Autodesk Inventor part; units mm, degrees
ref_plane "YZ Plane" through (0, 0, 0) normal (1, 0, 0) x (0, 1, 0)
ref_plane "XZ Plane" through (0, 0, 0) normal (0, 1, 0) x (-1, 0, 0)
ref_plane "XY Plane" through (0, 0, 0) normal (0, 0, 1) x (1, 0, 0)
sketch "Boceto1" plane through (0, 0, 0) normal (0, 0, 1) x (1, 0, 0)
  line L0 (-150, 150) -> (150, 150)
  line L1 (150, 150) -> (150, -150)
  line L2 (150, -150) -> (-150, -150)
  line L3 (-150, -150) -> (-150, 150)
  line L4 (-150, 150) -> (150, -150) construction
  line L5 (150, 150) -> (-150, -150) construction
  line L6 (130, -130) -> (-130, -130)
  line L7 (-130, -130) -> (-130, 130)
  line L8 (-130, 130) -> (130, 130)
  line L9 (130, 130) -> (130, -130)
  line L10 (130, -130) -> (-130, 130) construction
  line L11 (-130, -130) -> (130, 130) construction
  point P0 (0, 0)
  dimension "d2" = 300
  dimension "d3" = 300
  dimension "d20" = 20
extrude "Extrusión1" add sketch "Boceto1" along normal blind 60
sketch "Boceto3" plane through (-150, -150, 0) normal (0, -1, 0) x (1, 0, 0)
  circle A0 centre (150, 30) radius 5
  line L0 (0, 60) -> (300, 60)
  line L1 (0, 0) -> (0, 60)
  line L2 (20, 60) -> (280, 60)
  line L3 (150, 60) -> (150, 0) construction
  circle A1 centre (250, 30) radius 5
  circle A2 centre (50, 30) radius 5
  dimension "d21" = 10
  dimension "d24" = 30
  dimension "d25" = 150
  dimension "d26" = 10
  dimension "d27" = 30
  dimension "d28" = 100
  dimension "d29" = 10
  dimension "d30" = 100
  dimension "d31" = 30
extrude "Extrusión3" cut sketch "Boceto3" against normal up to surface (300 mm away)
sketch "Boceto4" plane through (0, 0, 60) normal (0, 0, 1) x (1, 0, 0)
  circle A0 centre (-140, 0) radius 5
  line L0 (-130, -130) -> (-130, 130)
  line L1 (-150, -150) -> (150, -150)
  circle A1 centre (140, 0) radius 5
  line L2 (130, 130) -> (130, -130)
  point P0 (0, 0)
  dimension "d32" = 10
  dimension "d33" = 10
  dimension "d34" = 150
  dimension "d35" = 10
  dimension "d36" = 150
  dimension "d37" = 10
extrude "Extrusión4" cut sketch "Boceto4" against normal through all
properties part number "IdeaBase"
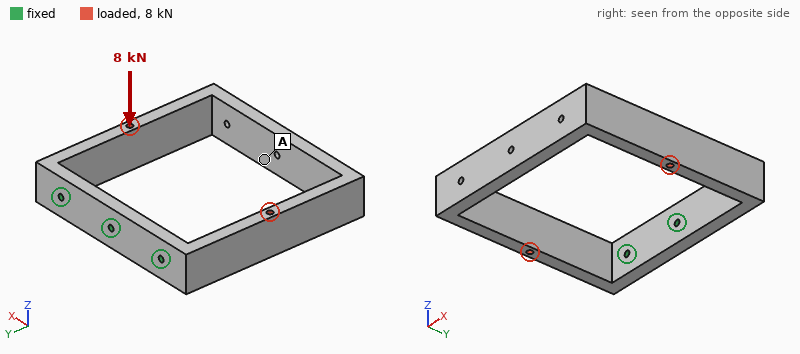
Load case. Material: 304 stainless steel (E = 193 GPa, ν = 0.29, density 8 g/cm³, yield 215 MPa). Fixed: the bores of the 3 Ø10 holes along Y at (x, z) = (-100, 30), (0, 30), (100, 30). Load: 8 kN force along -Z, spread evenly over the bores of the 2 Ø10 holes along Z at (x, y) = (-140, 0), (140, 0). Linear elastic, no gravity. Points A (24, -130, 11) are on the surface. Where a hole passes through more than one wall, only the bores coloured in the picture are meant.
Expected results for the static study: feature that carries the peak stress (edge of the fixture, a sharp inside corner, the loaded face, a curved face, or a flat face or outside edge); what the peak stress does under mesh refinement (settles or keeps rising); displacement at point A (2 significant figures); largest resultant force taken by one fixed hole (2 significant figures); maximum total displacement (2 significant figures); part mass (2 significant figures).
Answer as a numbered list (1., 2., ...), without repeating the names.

1. edge of the fixture
2. keeps rising
3. 0.68 mm
4. 5.4 kN
5. 0.74 mm
6. 11 kg
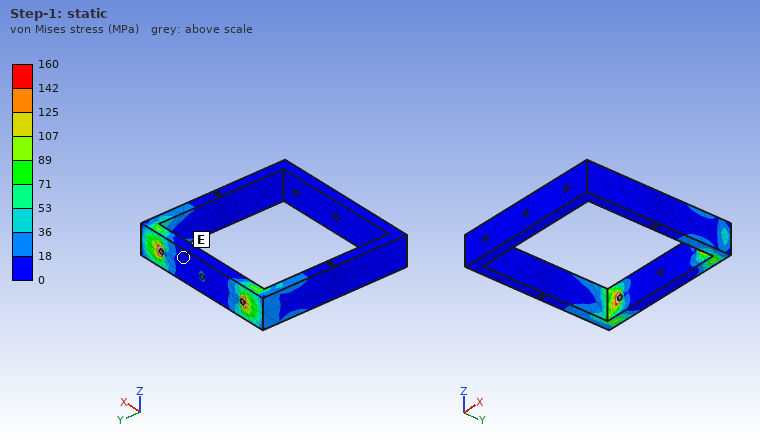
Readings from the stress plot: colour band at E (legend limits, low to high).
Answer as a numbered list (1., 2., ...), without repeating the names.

1. 0 to 18 MPa
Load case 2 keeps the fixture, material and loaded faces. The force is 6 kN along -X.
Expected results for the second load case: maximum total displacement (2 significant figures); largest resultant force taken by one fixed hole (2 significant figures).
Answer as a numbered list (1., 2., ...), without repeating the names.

1. 0.71 mm
2. 3.2 kN
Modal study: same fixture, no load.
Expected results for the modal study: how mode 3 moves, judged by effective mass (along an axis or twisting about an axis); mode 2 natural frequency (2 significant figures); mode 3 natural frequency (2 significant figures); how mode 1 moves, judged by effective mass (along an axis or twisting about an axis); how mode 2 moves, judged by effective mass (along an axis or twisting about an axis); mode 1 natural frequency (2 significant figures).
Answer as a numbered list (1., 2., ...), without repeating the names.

1. twisting about Y
2. 170 Hz
3. 320 Hz
4. along X
5. along Z
6. 150 Hz
